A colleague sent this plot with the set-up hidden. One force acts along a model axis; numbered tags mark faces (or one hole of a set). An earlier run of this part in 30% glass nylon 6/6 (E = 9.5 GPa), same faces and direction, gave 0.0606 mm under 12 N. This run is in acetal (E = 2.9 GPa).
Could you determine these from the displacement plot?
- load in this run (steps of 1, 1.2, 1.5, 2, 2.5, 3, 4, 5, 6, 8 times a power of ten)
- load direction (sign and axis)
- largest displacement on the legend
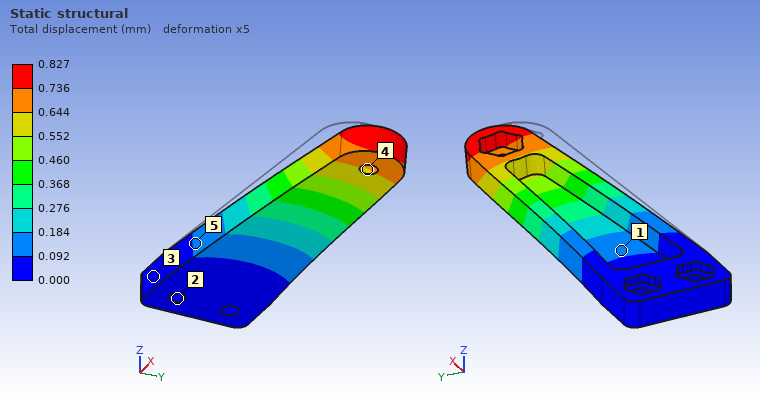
50 N
+Y
0.827 mm
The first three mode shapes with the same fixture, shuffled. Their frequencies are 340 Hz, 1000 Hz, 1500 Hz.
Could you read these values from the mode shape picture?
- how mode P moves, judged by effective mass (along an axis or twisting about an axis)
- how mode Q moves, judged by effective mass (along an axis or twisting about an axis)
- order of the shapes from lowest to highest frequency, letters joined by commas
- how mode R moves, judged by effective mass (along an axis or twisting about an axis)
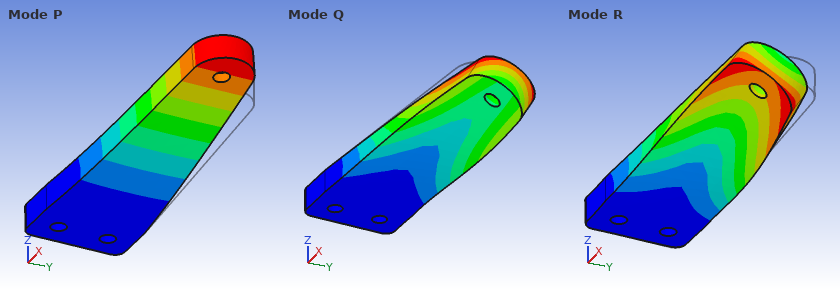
along Z
along Y
P, Q, R
along Y
